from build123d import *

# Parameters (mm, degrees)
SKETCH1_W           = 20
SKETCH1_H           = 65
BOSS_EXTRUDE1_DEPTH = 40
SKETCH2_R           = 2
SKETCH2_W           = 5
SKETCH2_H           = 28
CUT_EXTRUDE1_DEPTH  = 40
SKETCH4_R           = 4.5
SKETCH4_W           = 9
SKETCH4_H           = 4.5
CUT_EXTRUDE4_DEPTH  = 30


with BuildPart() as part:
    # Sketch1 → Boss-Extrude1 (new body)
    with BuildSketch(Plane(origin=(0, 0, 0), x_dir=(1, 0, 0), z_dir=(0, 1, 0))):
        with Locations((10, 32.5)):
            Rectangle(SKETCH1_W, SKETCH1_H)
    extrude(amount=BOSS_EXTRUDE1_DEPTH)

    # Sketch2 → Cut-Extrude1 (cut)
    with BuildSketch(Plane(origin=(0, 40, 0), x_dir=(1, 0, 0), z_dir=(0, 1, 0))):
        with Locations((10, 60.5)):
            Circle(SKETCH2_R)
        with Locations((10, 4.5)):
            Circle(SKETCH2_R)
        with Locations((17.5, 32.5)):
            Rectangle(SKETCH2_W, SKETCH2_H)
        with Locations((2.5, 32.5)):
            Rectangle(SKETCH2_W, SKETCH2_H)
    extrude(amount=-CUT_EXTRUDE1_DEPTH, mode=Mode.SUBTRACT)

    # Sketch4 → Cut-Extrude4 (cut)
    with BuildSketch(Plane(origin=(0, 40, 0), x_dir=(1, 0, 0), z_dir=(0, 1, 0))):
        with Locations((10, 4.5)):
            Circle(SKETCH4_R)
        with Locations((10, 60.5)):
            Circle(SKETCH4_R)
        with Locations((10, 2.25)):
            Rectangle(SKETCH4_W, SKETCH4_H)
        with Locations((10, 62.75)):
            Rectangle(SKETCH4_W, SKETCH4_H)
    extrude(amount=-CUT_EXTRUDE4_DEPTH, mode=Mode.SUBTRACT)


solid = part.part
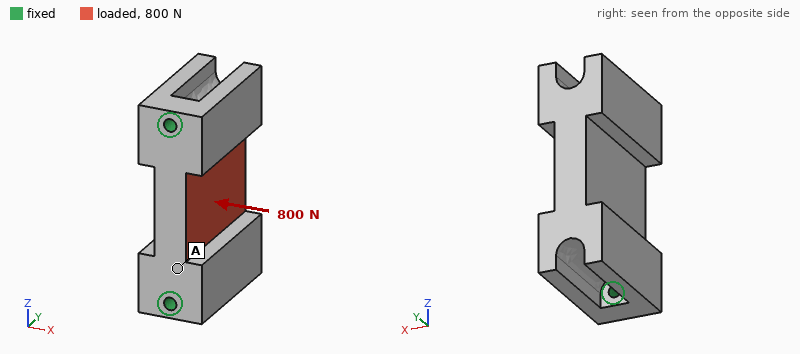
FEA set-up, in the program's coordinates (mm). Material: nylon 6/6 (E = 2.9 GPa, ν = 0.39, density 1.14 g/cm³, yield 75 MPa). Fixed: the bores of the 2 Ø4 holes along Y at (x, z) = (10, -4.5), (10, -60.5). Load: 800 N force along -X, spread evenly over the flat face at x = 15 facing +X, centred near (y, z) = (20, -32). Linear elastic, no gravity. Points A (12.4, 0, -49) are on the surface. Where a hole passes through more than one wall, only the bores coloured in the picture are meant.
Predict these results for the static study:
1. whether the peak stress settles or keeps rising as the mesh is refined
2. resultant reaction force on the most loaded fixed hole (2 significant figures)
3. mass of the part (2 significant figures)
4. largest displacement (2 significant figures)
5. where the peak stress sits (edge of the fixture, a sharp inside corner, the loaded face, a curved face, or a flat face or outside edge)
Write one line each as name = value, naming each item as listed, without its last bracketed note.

whether the peak stress settles or keeps rising as the mesh is refined = keeps rising
resultant reaction force on the most loaded fixed hole = 400 N
mass of the part = 41 g
largest displacement = 0.45 mm
where the peak stress sits = edge of the fixture
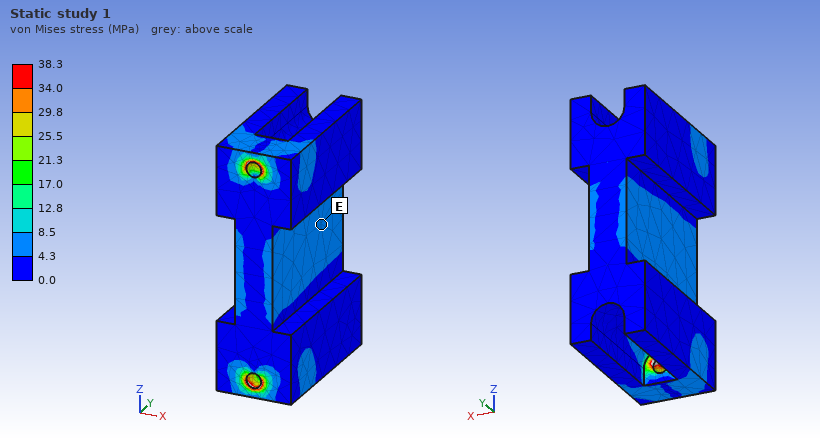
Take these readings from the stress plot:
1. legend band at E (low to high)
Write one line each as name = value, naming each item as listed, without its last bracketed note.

legend band at E = 4.3 to 8.5 MPa
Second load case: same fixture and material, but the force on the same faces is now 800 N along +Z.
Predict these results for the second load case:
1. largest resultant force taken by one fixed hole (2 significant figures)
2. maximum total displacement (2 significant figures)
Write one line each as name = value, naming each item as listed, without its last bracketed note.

largest resultant force taken by one fixed hole = 460 N
maximum total displacement = 62 µm
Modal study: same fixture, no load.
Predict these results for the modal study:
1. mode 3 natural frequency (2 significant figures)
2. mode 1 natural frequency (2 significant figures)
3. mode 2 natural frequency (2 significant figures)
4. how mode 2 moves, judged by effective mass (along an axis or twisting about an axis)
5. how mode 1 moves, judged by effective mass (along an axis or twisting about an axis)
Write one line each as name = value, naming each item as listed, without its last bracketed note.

mode 3 natural frequency = 3500 Hz
mode 1 natural frequency = 1400 Hz
mode 2 natural frequency = 2500 Hz
how mode 2 moves, judged by effective mass = twisting about Y
how mode 1 moves, judged by effective mass = along X
